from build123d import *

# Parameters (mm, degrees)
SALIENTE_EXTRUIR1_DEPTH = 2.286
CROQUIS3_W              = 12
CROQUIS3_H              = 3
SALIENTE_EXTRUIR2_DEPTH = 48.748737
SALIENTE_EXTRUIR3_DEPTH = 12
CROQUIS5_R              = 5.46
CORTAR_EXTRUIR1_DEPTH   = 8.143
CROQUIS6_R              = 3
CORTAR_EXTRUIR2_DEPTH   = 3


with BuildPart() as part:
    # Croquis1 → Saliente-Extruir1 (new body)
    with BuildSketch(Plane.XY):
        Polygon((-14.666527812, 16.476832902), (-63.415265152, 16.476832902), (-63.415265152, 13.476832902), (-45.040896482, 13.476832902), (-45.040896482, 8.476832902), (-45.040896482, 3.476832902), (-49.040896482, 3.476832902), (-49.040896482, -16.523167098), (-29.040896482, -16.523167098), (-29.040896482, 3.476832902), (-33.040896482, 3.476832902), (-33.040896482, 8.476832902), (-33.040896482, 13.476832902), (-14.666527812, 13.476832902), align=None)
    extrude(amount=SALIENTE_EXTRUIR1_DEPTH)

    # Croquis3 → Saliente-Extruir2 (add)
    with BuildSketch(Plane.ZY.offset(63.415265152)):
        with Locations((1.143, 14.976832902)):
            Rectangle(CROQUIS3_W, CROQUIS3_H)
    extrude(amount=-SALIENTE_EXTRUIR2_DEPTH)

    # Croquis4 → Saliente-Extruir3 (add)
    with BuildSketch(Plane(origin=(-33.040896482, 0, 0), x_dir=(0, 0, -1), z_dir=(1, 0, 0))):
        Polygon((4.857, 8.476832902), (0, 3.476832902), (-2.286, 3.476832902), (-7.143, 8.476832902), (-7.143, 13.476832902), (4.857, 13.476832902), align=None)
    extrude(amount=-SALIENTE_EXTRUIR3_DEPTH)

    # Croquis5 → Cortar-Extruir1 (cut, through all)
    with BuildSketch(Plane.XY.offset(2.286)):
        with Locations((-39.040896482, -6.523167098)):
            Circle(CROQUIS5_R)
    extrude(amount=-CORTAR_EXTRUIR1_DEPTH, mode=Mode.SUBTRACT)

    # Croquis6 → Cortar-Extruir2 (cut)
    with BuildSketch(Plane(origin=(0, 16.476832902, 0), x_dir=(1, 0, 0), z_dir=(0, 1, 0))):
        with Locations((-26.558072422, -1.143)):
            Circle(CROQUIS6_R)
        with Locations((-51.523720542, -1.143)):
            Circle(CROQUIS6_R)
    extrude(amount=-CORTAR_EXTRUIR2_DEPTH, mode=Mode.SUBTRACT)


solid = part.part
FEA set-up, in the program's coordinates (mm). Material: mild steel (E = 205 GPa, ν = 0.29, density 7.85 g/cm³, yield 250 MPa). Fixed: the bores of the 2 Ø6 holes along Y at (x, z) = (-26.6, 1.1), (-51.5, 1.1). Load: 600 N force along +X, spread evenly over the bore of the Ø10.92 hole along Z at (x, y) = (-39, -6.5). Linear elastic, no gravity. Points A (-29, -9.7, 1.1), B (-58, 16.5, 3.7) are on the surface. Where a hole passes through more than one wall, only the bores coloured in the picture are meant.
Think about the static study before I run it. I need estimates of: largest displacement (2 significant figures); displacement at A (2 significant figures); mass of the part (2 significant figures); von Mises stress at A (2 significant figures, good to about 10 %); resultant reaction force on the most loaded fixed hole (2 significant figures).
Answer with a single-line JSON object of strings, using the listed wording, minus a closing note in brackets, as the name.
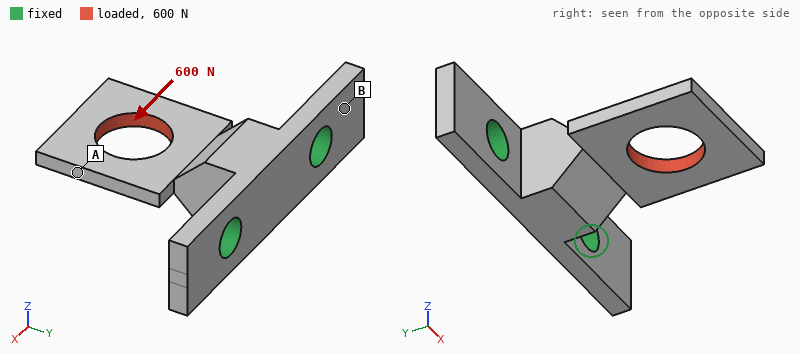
{"largest displacement": "50 µm", "displacement at A": "40 µm", "mass of the part": "27 g", "von Mises stress at A": "40 MPa", "resultant reaction force on the most loaded fixed hole": "840 N"}
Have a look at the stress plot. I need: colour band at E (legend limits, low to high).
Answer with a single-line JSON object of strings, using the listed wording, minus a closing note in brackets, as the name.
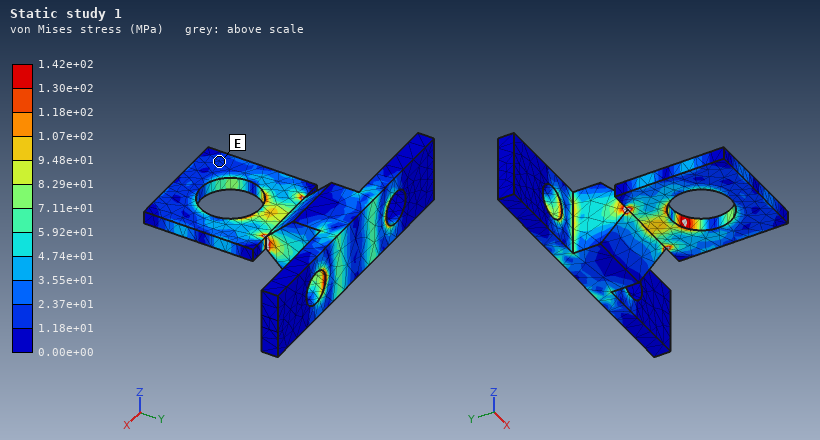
{"colour band at E": "1.18e+01 to 2.37e+01 MPa"}
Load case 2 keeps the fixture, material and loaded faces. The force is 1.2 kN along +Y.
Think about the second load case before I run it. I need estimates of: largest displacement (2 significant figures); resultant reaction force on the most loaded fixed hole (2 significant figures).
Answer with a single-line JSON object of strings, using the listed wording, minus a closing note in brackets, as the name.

{"largest displacement": "11 µm", "resultant reaction force on the most loaded fixed hole": "650 N"}
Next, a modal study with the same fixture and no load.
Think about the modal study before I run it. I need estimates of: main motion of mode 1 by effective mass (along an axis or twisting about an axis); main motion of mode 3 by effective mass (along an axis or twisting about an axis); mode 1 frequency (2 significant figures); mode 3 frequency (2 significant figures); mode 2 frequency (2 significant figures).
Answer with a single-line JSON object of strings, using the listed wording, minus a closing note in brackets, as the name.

{"main motion of mode 1 by effective mass": "along Z", "main motion of mode 3 by effective mass": "along X", "mode 1 frequency": "3100 Hz", "mode 3 frequency": "8400 Hz", "mode 2 frequency": "7600 Hz"}
